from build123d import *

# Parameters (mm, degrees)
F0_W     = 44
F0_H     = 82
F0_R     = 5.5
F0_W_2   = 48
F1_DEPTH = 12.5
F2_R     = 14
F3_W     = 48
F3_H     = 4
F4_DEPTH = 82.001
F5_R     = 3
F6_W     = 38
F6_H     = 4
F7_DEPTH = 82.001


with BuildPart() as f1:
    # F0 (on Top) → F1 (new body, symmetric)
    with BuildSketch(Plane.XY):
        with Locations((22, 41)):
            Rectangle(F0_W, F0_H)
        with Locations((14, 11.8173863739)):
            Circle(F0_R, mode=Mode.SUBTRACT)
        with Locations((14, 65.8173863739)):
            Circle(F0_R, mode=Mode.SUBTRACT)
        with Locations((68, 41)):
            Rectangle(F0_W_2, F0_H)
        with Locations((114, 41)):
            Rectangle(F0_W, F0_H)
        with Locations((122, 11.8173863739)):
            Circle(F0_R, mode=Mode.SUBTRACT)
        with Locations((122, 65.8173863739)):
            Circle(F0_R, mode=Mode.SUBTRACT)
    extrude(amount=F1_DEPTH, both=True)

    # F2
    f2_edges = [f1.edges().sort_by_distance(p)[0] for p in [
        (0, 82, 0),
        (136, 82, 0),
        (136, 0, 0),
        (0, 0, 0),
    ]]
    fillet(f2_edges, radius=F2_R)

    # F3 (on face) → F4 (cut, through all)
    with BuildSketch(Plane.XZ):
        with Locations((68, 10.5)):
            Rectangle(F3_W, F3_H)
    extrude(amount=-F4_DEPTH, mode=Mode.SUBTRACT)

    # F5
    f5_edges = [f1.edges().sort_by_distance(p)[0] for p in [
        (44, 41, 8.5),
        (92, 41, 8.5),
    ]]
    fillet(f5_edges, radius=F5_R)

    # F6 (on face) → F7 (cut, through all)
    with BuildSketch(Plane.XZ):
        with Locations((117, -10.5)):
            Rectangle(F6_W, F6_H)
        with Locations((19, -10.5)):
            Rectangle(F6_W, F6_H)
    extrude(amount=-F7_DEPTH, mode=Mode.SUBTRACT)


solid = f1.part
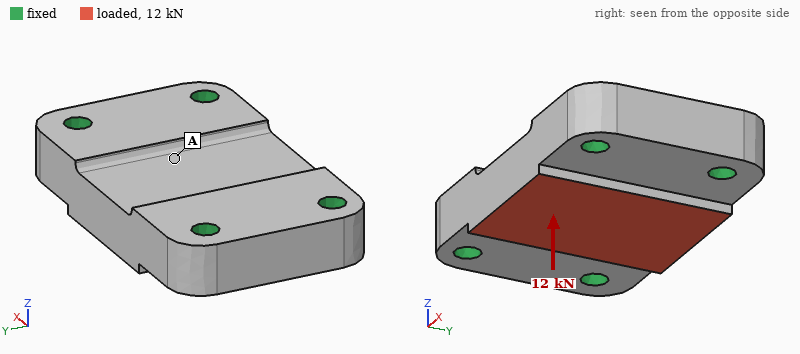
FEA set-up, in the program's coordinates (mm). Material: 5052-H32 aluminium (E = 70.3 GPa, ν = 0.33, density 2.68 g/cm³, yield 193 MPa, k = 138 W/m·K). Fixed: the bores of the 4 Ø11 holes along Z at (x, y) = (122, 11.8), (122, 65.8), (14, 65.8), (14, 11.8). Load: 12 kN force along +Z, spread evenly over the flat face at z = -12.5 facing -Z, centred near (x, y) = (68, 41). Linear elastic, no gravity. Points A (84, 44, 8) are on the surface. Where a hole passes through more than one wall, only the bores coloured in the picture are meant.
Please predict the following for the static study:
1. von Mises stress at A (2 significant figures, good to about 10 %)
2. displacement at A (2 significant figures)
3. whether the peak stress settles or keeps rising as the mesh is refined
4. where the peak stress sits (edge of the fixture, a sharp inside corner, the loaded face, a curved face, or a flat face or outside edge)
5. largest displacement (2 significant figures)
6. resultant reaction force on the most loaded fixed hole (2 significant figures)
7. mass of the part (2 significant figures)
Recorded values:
7.9 MPa
16 µm
keeps rising
edge of the fixture
20 µm
3.6 kN
610 g
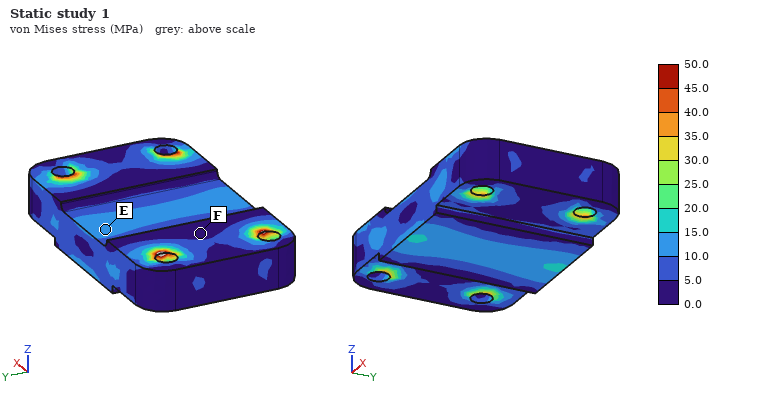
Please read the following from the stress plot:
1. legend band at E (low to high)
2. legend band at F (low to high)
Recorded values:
10.0 to 15.0 MPa
0.0 to 5.0 MPa
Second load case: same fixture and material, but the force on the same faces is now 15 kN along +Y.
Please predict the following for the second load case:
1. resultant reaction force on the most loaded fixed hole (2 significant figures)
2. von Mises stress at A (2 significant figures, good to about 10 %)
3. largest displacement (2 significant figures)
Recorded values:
5.2 kN
2.7 MPa
21 µm
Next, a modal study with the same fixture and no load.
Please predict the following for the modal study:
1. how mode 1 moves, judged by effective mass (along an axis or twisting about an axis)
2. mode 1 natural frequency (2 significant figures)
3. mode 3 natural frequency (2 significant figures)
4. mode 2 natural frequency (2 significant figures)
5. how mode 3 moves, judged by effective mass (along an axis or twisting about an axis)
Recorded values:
along Z
7700 Hz
13 kHz
9900 Hz
along Y
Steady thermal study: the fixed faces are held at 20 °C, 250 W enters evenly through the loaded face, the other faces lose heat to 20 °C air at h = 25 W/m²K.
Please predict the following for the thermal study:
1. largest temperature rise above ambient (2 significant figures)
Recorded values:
24 K
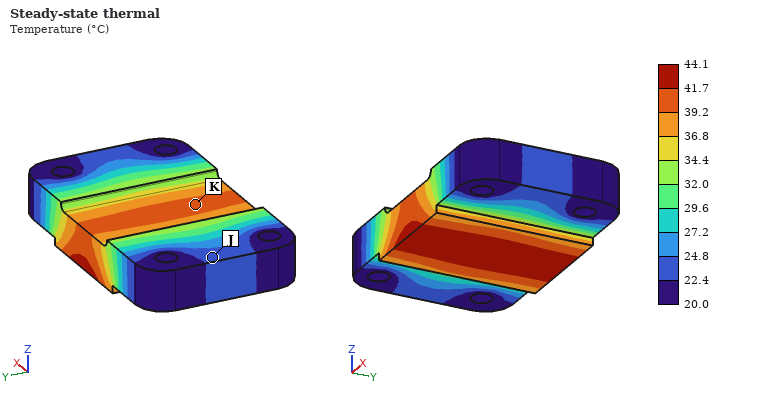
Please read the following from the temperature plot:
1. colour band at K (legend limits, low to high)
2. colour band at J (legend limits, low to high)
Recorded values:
39.2 to 41.7 °C
22.4 to 24.8 °C
